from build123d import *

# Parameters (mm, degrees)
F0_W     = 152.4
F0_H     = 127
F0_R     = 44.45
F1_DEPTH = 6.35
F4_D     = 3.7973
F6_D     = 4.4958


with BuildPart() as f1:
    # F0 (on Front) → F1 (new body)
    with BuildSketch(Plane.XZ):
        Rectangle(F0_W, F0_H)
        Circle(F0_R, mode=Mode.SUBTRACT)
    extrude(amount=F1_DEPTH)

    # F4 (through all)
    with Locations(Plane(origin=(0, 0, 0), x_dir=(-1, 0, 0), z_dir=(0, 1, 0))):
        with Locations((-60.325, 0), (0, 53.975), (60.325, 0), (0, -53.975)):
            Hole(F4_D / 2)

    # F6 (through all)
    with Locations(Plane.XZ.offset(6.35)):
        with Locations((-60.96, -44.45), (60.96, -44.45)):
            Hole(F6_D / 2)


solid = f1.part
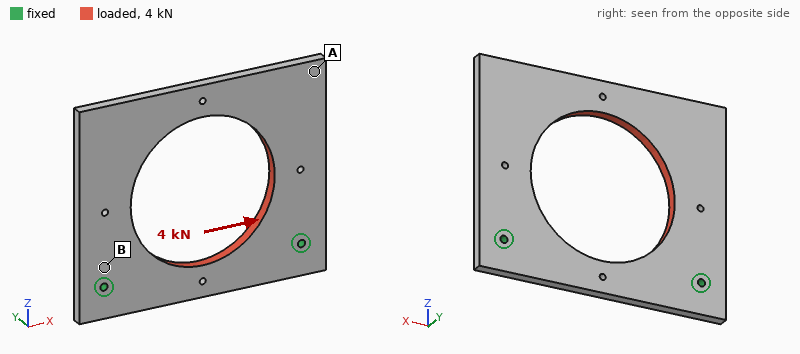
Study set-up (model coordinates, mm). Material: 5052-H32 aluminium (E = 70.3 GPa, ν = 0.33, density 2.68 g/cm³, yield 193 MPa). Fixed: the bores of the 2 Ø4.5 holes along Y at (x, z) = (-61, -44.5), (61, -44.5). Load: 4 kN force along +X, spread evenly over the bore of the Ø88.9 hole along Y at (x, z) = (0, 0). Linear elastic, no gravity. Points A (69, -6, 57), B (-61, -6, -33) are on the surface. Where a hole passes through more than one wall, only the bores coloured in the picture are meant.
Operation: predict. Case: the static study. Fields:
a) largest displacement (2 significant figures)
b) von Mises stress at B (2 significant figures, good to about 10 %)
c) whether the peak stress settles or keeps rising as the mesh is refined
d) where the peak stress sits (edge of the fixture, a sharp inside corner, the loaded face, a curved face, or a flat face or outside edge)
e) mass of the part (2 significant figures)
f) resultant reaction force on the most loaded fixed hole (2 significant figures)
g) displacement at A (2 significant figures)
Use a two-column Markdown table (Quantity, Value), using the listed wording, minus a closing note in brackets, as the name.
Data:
| Quantity | Value |
|---|---|
| largest displacement | 92 µm |
| von Mises stress at B | 12 MPa |
| whether the peak stress settles or keeps rising as the mesh is refined | keeps rising |
| where the peak stress sits | edge of the fixture |
| mass of the part | 220 g |
| resultant reaction force on the most loaded fixed hole | 2.4 kN |
| displacement at A | 88 µm |
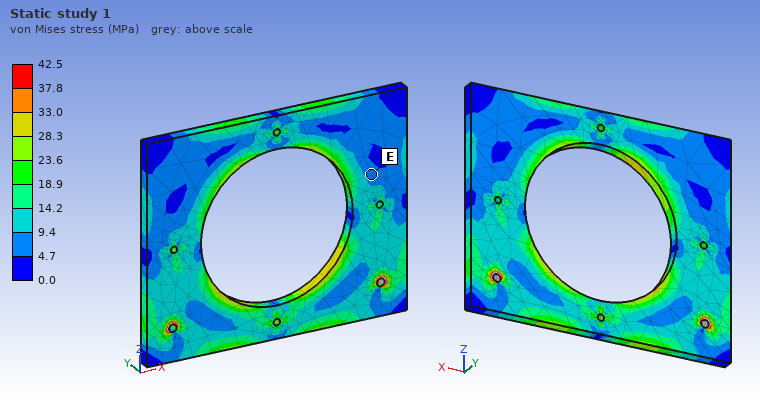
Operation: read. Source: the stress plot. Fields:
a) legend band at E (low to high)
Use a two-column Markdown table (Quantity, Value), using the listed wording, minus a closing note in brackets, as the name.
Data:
| Quantity | Value |
|---|---|
| legend band at E | 4.7 to 9.4 MPa |
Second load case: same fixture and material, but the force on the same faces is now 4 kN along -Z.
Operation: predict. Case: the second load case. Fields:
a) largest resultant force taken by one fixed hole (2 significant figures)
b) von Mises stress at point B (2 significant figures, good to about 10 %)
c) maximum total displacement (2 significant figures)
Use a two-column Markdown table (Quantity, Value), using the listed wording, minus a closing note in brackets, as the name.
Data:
| Quantity | Value |
|---|---|
| largest resultant force taken by one fixed hole | 2.0 kN |
| von Mises stress at point B | 13 MPa |
| maximum total displacement | 17 µm |
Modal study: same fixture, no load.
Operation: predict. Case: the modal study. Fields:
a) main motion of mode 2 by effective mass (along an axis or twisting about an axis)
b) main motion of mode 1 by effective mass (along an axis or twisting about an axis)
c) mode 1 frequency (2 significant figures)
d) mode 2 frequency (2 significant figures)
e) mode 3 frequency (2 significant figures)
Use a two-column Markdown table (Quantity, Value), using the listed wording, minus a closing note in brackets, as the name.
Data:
| Quantity | Value |
|---|---|
| main motion of mode 2 by effective mass | twisting about Z |
| main motion of mode 1 by effective mass | along Y |
| mode 1 frequency | 330 Hz |
| mode 2 frequency | 680 Hz |
| mode 3 frequency | 1700 Hz |
